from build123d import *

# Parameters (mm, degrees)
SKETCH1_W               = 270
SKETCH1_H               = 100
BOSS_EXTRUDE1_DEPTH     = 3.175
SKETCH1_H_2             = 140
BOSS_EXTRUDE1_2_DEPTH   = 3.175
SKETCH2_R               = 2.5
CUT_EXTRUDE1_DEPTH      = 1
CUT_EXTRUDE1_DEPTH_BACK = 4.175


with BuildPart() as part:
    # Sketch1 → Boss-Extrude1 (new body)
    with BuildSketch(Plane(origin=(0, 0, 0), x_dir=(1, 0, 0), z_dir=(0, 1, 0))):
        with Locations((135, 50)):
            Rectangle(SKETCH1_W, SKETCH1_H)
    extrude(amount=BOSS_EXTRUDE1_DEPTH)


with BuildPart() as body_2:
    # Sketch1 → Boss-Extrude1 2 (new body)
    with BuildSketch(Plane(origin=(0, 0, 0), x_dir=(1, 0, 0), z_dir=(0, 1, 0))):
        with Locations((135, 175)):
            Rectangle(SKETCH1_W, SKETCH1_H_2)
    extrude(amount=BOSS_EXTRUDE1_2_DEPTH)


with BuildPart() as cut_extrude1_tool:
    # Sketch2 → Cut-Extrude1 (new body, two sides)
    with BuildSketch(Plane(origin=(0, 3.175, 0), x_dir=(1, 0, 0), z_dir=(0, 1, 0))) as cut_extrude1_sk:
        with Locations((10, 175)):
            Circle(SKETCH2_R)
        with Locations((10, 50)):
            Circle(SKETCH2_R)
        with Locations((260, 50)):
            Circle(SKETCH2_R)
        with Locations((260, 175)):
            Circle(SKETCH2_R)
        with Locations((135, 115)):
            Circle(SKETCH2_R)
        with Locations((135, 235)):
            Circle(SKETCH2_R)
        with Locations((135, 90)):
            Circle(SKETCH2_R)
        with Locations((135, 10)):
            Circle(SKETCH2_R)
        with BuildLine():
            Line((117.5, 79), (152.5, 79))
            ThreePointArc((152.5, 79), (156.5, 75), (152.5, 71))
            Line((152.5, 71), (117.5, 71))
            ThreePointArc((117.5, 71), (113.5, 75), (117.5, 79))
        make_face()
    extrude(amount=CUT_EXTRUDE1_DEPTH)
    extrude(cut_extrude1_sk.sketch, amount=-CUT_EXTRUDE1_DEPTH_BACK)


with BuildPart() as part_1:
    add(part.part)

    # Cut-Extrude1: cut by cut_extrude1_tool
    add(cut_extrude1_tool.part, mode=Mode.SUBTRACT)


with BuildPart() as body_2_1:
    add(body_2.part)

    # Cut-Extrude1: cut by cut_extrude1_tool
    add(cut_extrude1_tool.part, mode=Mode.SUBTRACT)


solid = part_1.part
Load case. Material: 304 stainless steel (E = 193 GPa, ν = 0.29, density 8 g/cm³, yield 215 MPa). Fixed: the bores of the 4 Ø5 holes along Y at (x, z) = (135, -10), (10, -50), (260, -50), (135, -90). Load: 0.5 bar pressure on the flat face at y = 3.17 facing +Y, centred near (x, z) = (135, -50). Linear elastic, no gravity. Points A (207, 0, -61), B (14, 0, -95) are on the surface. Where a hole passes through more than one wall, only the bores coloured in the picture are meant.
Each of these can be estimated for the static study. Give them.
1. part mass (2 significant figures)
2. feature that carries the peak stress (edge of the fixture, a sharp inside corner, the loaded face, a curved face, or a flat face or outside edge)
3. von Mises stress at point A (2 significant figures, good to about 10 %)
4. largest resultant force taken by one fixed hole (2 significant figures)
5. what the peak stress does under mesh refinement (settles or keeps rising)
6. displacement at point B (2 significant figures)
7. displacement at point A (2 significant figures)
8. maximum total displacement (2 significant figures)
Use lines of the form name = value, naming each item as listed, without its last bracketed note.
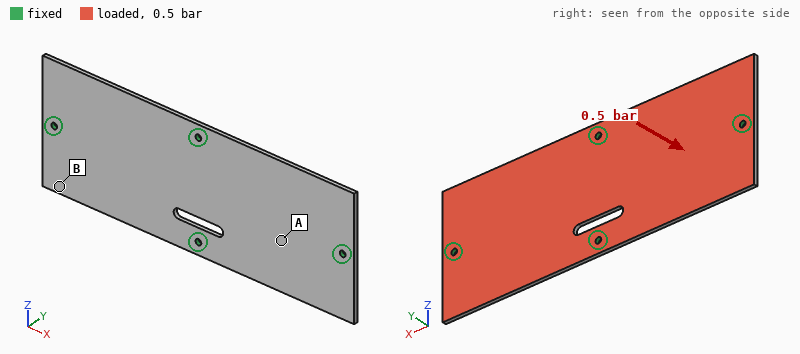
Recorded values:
part mass = 680 g
feature that carries the peak stress = edge of the fixture
von Mises stress at point A = 22 MPa
largest resultant force taken by one fixed hole = 350 N
what the peak stress does under mesh refinement = keeps rising
displacement at point B = 0.069 mm
displacement at point A = 0.090 mm
maximum total displacement = 0.12 mm
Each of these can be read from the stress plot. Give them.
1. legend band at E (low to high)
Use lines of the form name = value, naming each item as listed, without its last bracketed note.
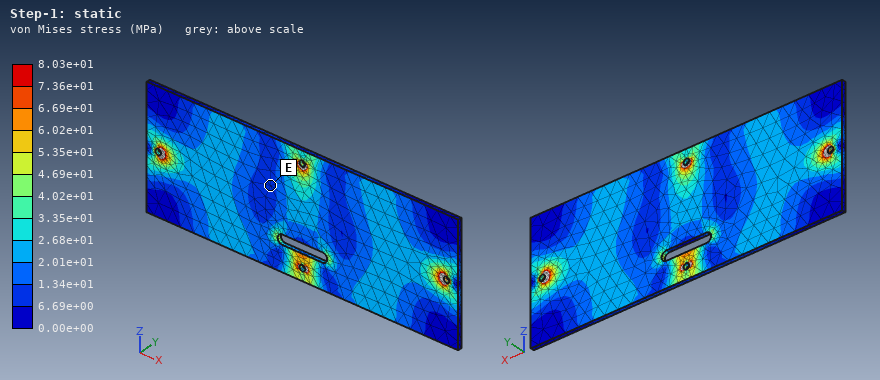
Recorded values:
legend band at E = 6.69e+00 to 1.34e+01 MPa
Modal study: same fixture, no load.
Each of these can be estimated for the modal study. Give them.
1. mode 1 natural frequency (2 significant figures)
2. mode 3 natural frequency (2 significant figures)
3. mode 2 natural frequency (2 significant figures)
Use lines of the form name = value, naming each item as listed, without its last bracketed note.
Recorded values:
mode 1 natural frequency = 750 Hz
mode 3 natural frequency = 770 Hz
mode 2 natural frequency = 770 Hz
